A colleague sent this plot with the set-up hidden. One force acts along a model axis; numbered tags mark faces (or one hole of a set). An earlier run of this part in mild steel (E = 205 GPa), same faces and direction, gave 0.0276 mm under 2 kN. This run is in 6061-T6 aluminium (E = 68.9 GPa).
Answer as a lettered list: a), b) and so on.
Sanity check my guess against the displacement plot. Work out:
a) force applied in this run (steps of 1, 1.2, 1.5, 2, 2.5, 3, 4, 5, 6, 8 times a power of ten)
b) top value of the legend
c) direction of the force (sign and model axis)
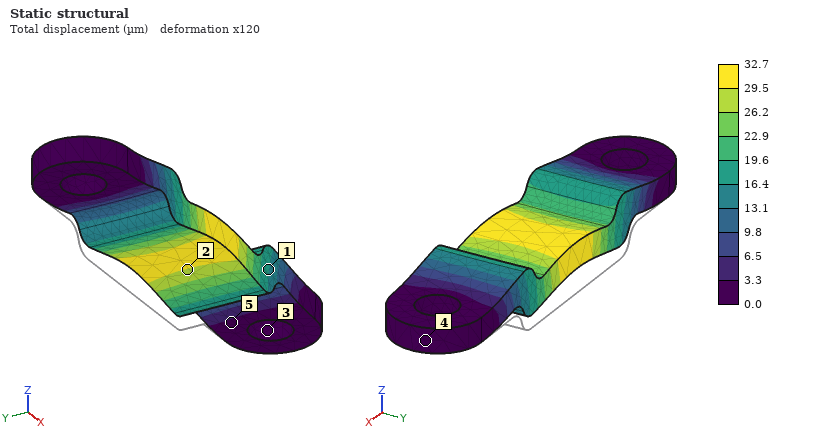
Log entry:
a) 800 N
b) 32.7 µm
c) +Z
